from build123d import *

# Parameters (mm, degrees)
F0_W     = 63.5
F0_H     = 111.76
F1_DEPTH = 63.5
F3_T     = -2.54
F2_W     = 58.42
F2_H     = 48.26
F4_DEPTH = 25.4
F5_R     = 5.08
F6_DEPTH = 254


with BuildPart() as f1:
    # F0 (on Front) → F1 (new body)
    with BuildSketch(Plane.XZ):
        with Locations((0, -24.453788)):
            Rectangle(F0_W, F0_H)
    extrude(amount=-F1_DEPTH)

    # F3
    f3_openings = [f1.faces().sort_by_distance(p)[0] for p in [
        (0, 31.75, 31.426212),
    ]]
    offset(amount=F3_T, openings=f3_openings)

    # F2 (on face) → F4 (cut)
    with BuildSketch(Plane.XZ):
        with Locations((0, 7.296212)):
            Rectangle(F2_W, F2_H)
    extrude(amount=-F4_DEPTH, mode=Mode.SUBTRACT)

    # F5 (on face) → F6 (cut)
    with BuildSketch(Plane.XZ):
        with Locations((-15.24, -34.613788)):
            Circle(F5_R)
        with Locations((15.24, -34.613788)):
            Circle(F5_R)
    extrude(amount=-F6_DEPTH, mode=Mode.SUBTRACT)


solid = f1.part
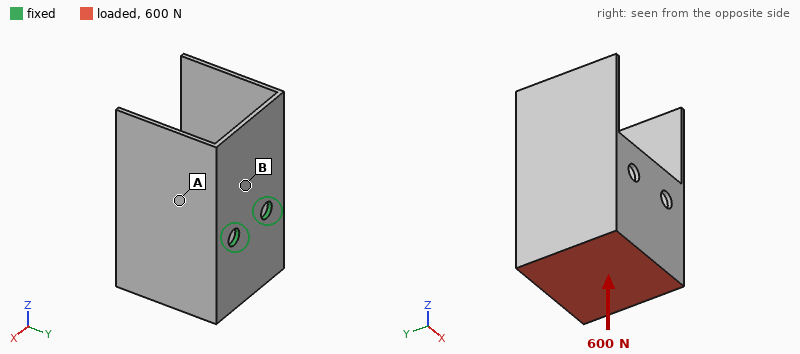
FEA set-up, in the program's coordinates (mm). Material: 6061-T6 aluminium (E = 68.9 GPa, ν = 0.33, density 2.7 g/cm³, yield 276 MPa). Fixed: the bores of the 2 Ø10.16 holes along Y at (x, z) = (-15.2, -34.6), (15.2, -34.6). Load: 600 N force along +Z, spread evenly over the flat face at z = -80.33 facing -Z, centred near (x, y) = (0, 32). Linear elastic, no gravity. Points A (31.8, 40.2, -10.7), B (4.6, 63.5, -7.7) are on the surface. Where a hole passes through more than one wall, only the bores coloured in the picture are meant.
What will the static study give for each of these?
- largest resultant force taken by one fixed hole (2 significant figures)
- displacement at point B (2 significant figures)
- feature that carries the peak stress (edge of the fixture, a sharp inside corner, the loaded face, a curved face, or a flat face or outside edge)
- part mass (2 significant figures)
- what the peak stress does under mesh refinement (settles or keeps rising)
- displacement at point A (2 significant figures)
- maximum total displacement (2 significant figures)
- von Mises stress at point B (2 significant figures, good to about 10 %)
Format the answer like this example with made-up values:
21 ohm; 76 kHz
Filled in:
300 N; 0.14 mm; edge of the fixture; 190 g; keeps rising; 0.26 mm; 0.72 mm; 19 MPa
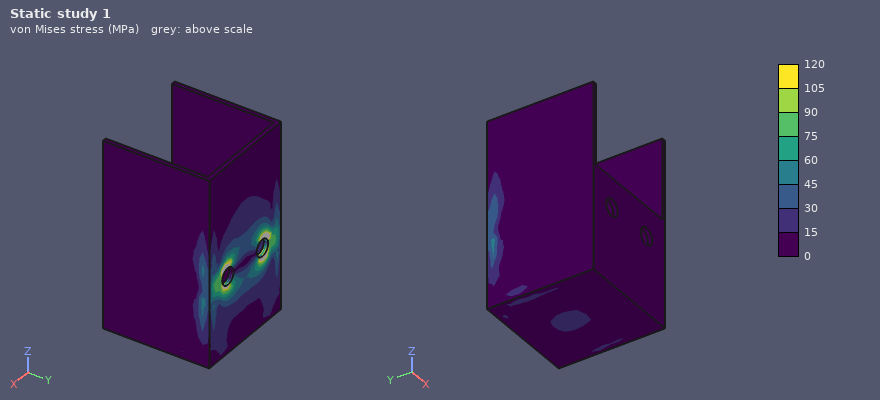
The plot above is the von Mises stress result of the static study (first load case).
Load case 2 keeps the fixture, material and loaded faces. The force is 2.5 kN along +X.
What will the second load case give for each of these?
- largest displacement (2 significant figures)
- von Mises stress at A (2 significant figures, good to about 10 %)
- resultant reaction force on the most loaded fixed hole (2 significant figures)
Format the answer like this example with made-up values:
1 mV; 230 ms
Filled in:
1.7 mm; 26 MPa; 3.5 kN
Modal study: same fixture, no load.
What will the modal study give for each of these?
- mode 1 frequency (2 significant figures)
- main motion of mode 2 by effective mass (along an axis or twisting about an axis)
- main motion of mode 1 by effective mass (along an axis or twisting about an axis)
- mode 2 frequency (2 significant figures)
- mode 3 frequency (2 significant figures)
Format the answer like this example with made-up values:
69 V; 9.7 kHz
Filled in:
360 Hz; along X; along Z; 470 Hz; 1000 Hz
